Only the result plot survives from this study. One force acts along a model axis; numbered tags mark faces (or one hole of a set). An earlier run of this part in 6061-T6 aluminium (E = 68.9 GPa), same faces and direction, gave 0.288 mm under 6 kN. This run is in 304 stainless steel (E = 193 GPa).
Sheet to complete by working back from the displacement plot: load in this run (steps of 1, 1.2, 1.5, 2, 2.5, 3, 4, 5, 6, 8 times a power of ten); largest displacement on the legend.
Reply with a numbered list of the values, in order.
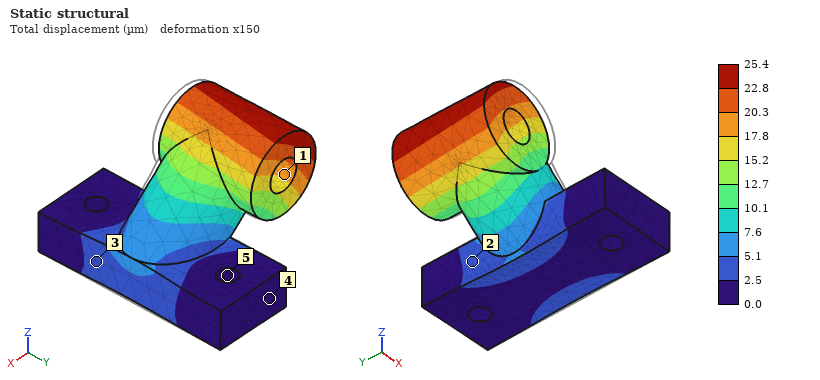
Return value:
1. 1.5 kN
2. 25.4 µm
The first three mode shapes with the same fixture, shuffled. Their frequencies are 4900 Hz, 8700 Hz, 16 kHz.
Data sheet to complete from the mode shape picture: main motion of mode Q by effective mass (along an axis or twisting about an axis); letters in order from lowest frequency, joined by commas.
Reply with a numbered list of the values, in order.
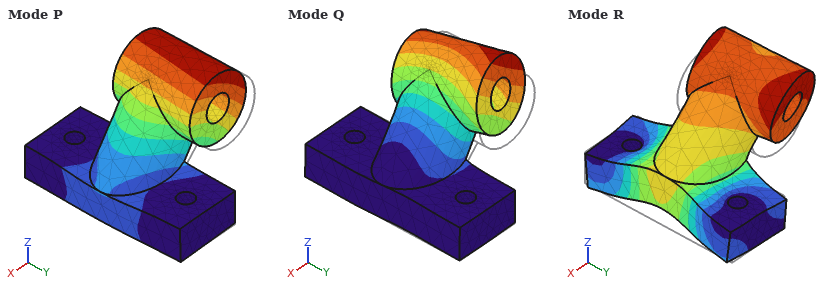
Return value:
1. along Y
2. P, Q, R
